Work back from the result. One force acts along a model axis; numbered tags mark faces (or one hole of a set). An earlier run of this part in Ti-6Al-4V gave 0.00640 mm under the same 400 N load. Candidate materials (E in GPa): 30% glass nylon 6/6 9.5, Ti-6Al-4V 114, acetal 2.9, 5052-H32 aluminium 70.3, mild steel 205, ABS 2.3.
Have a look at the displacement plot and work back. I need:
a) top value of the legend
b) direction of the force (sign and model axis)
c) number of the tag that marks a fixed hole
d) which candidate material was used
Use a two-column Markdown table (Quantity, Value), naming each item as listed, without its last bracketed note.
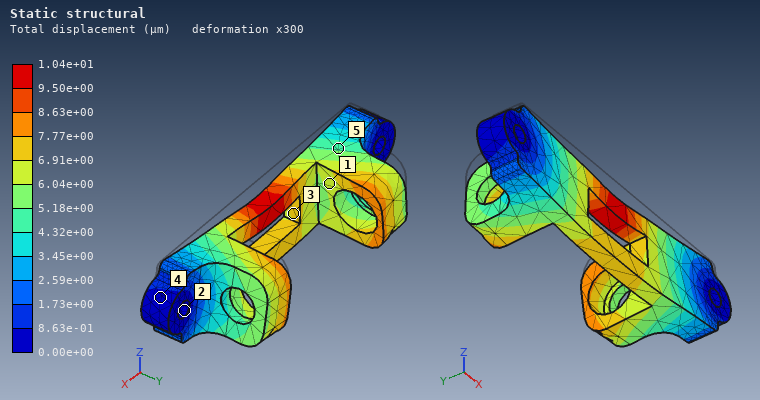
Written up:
| Quantity | Value |
|---|---|
| top value of the legend | 1.04e+01 µm |
| direction of the force | -Z |
| number of the tag that marks a fixed hole | 2 |
| which candidate material was used | 5052-H32 aluminium |
